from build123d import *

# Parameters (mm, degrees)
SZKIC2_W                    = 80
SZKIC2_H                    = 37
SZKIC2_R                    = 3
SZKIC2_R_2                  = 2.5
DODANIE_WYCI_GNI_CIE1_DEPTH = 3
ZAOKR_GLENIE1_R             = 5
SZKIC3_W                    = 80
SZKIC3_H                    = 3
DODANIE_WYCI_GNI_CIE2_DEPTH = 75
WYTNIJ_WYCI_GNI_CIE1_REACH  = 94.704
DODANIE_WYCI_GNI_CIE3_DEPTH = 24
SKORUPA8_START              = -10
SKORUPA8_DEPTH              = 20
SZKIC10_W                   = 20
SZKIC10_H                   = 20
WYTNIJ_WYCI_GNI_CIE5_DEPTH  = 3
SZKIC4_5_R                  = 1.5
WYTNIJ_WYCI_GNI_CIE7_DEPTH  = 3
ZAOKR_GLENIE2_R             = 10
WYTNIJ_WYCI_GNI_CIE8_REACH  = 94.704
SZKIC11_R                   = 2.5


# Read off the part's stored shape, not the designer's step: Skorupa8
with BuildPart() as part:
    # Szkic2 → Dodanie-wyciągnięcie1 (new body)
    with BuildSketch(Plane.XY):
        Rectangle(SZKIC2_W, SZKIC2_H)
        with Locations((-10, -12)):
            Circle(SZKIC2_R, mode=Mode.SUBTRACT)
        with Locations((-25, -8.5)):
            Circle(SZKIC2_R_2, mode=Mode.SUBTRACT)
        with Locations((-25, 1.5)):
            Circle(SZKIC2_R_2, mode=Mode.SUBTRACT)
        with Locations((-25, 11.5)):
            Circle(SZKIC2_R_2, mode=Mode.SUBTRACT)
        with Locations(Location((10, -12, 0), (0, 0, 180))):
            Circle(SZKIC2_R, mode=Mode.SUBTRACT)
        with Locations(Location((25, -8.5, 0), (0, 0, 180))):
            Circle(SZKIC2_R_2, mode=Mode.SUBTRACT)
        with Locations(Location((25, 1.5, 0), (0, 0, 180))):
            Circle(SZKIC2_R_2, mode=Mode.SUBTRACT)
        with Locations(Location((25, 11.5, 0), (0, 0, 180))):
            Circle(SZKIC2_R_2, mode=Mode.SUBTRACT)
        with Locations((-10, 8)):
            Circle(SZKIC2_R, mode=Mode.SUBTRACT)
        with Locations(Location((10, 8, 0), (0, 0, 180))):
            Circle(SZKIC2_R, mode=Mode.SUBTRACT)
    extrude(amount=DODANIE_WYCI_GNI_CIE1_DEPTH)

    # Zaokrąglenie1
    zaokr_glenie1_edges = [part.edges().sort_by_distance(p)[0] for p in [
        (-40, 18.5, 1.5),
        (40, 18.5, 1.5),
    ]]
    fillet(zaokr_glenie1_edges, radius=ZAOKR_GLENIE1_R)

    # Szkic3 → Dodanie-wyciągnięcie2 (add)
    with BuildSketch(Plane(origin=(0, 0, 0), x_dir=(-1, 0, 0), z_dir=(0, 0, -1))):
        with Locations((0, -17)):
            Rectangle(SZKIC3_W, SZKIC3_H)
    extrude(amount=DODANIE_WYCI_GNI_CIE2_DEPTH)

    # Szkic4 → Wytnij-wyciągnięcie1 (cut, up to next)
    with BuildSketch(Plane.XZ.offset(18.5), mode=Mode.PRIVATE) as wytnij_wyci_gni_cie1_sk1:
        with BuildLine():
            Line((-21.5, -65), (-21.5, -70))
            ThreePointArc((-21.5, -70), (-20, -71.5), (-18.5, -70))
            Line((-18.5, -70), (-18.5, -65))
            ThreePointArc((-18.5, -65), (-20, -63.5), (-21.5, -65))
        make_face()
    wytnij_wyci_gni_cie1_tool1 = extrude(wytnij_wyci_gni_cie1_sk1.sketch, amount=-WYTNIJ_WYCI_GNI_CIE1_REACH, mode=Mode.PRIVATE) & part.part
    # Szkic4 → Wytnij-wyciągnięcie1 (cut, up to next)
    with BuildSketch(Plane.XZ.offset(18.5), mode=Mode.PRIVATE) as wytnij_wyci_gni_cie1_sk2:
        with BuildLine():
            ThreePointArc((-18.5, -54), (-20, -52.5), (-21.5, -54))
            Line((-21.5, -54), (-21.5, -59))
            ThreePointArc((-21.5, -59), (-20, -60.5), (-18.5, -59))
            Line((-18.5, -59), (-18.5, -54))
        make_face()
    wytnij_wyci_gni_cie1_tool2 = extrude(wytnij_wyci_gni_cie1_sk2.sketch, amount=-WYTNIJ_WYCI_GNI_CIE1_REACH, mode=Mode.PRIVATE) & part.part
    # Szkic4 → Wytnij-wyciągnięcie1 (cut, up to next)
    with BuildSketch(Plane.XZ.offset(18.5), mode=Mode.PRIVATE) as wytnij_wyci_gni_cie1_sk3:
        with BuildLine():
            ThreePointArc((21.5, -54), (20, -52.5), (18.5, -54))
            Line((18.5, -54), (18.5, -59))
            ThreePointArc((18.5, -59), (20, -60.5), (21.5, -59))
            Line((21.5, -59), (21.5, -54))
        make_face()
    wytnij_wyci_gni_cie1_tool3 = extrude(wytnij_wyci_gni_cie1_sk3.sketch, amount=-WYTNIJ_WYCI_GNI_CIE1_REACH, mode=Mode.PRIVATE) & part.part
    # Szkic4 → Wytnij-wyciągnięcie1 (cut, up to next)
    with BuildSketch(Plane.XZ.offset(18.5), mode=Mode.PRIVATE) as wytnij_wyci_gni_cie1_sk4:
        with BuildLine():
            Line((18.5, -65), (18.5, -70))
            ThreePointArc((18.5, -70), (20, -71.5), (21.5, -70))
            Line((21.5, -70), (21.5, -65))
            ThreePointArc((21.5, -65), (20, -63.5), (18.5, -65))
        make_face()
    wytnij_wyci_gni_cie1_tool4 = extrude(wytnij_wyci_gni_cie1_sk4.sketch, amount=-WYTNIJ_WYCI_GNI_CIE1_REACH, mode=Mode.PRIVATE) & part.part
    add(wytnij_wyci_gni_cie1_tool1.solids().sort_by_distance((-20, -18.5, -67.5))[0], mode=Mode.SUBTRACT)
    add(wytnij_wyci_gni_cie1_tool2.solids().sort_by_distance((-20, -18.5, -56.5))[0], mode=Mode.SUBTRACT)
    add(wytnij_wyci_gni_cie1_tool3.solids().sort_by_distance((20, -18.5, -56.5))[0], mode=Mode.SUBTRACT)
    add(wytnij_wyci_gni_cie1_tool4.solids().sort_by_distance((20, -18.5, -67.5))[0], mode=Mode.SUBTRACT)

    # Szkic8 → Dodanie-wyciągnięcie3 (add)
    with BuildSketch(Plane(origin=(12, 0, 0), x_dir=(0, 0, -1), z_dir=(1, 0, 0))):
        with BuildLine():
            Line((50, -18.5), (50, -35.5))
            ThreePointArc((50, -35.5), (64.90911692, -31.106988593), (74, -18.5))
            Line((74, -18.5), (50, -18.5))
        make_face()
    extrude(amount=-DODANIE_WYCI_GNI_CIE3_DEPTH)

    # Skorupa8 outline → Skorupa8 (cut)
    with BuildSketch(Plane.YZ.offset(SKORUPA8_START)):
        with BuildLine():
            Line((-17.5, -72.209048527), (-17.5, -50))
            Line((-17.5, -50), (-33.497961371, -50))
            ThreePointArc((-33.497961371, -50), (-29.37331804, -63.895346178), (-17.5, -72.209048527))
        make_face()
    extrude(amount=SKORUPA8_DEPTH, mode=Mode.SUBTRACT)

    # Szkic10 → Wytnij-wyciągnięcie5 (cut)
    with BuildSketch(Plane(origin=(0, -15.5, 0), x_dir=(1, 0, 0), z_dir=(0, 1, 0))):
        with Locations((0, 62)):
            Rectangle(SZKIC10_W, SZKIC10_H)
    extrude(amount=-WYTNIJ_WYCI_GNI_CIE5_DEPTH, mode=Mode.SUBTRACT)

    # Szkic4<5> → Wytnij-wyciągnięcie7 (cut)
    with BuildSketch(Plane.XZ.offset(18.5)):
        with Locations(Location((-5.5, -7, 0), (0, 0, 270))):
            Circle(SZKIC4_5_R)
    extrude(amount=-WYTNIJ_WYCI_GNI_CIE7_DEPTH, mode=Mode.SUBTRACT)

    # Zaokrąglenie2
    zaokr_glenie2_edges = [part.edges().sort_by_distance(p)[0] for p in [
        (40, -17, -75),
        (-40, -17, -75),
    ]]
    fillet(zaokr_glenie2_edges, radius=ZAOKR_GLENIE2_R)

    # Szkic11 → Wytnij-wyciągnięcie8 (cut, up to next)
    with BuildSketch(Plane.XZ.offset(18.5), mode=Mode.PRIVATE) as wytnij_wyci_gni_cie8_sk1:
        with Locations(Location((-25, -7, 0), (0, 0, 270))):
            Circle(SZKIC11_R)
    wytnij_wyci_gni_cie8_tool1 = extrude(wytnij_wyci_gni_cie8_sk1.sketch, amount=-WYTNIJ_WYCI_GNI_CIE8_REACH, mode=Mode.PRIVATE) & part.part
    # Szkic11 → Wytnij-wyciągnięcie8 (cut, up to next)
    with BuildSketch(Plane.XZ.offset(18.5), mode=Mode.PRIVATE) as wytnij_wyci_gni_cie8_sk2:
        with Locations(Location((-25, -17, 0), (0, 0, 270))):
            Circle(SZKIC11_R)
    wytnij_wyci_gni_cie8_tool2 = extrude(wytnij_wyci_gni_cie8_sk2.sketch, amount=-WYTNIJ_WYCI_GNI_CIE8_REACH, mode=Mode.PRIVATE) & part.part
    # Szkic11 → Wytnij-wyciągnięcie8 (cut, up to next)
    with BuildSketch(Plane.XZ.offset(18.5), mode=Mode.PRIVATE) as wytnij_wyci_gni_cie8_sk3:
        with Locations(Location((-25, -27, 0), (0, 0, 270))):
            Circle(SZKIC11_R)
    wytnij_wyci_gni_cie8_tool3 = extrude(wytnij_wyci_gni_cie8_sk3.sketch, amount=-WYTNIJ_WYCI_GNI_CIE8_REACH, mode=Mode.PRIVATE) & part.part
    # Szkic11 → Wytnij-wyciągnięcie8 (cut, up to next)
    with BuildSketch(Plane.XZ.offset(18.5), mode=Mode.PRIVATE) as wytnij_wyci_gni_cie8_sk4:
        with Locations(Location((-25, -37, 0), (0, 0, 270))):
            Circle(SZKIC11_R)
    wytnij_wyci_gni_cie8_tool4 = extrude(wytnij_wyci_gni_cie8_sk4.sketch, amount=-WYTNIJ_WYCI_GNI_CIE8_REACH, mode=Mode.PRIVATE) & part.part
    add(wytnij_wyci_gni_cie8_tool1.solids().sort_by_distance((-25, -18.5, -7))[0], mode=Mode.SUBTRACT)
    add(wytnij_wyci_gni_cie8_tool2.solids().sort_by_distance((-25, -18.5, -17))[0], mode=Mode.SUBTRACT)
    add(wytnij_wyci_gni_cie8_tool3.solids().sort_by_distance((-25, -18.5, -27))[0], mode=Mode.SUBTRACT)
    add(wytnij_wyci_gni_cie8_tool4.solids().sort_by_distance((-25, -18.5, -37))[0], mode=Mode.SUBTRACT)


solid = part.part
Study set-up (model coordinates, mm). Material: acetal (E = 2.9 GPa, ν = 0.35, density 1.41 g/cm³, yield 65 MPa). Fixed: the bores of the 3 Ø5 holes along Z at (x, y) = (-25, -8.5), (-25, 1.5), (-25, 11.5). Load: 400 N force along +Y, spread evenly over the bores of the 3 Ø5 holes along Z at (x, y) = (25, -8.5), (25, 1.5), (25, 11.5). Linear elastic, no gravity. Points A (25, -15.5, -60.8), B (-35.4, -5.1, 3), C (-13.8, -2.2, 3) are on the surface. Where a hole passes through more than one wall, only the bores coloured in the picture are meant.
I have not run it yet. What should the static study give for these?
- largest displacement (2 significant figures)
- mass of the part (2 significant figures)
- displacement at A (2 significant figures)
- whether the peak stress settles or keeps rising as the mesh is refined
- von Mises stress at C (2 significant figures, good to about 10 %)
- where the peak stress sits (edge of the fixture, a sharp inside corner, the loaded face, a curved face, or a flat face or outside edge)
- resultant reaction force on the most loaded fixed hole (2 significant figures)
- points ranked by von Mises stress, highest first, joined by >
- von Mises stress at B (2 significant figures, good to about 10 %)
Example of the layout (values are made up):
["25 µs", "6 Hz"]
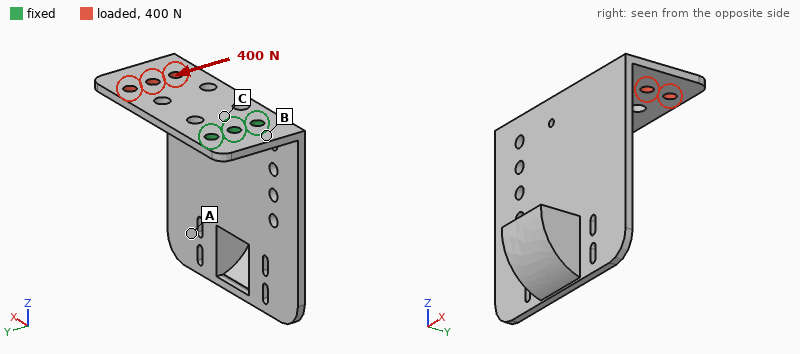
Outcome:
["1.00 mm", "38 g", "0.65 mm", "keeps rising", "12 MPa", "edge of the fixture", "890 N", "C > B > A", "5.1 MPa"]
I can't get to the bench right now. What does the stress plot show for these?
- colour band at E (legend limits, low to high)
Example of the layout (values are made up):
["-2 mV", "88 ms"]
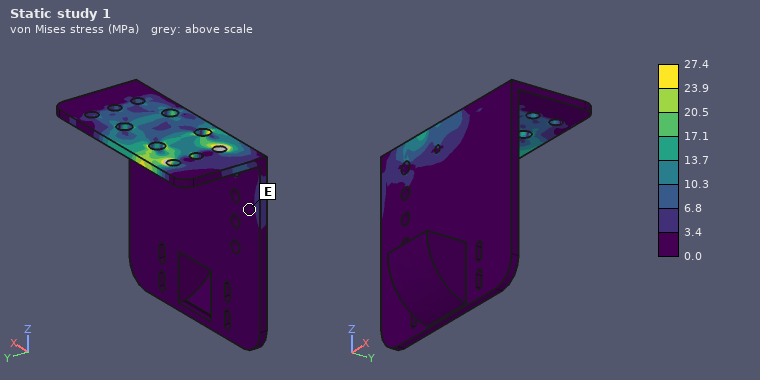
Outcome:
["0.0 to 3.4 MPa"]
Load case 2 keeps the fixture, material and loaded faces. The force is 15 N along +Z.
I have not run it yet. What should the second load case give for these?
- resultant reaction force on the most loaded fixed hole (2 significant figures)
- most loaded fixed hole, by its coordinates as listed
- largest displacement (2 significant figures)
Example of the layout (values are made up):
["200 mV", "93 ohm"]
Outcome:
["6.0 N", "(-25, 1.5)", "1.1 mm"]
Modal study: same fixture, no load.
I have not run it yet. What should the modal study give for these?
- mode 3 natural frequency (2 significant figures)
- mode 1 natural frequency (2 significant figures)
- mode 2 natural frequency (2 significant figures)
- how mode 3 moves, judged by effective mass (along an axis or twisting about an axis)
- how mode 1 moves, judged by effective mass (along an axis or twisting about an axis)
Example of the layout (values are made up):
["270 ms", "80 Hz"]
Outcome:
["250 Hz", "78 Hz", "130 Hz", "twisting about Z", "along Y"]
